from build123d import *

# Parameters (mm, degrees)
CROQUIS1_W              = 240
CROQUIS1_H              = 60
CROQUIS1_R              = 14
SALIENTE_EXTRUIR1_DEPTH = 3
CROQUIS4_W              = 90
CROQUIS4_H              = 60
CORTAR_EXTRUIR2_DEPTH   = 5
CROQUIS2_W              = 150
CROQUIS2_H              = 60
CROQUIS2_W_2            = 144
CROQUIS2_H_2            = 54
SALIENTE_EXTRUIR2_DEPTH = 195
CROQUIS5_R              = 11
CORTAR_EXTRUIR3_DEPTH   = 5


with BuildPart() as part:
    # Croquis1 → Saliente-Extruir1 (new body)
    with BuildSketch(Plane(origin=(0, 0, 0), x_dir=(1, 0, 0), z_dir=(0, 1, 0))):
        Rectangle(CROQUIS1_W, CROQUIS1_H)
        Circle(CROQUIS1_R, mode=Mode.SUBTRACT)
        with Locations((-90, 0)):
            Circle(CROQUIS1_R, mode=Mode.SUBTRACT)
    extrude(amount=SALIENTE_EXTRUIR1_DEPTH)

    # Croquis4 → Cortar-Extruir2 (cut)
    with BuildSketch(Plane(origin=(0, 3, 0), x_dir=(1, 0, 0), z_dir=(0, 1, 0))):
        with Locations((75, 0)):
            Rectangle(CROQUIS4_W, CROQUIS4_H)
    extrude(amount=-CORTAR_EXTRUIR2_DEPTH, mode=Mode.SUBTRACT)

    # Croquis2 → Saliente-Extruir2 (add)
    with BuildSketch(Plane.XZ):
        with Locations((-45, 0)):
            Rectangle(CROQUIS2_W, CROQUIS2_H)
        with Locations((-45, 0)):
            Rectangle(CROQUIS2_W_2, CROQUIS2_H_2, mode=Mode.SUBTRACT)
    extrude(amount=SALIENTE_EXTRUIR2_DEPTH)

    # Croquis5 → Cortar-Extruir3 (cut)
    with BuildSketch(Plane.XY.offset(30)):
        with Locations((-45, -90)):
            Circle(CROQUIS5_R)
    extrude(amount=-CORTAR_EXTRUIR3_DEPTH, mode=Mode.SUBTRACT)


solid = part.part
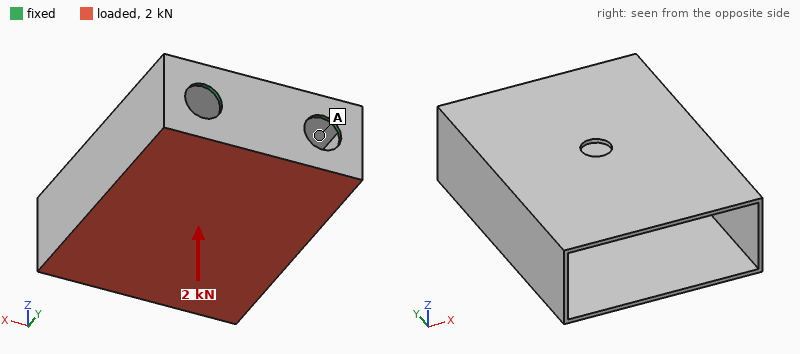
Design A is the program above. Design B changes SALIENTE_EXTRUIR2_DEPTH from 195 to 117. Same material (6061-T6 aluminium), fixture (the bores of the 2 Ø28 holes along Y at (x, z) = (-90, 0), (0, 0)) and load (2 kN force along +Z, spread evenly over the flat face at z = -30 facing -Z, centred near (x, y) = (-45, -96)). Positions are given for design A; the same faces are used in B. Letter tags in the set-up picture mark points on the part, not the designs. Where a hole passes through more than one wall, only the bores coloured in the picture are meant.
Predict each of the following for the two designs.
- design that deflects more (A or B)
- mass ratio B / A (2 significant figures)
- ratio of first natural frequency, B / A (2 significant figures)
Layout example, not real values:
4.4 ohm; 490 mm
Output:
A; 0.63; 1.8
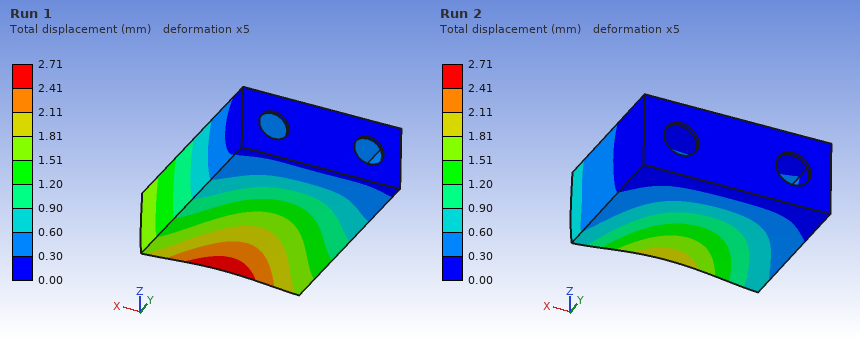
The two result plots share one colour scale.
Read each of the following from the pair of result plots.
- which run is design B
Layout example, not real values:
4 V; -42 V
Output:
Run 2
